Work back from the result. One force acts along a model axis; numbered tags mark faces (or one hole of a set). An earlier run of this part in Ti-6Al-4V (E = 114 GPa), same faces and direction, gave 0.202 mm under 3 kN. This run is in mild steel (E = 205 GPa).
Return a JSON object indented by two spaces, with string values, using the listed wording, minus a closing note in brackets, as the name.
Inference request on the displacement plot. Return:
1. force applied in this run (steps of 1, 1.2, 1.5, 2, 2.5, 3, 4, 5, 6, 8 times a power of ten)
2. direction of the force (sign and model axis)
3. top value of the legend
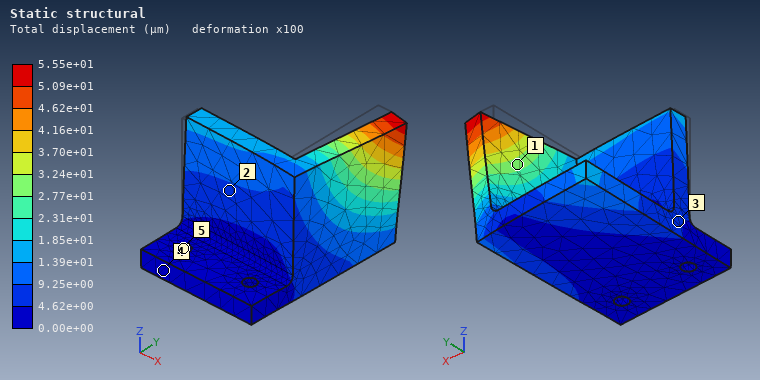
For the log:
{
  "force applied in this run": "1.5 kN",
  "direction of the force": "+X",
  "top value of the legend": "5.55e+01 µm"
}
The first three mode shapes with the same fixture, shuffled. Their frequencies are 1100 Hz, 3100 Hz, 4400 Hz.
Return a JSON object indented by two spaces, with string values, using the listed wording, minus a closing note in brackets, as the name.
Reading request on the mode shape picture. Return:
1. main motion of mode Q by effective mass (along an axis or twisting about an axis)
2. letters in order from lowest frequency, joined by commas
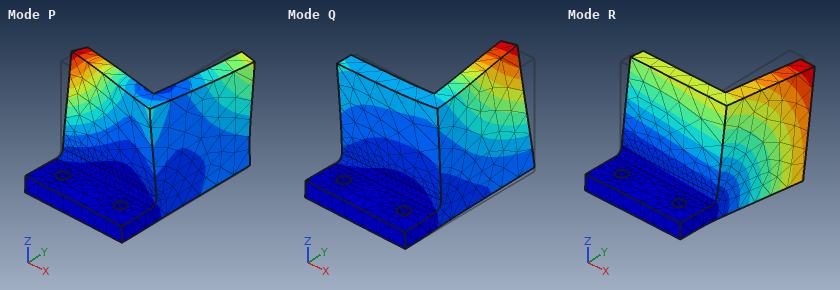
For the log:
{
  "main motion of mode Q by effective mass": "along X",
  "letters in order from lowest frequency, joined by commas": "R, Q, P"
}
